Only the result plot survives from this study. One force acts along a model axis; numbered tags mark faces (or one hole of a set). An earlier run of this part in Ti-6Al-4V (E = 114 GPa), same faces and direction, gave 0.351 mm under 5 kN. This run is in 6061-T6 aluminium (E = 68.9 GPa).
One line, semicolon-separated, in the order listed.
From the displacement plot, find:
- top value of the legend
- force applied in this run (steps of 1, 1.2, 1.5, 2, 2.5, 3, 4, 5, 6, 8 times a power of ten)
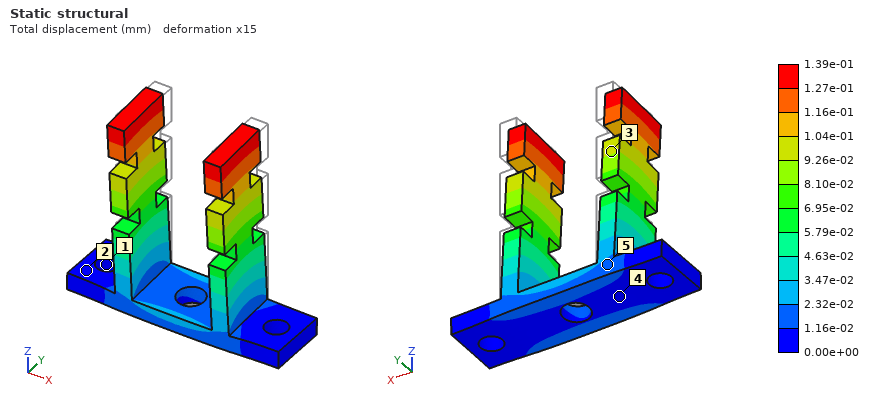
1.39e-01 mm; 1.2 kN
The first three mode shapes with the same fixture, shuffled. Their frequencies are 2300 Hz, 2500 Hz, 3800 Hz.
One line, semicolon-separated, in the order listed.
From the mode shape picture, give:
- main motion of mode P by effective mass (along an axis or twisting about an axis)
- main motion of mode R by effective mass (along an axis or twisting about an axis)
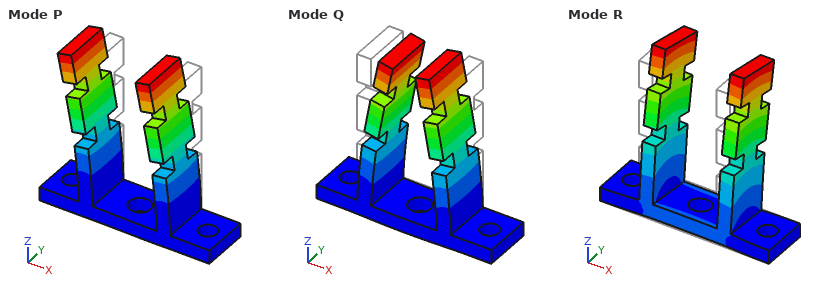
along X; along Y
